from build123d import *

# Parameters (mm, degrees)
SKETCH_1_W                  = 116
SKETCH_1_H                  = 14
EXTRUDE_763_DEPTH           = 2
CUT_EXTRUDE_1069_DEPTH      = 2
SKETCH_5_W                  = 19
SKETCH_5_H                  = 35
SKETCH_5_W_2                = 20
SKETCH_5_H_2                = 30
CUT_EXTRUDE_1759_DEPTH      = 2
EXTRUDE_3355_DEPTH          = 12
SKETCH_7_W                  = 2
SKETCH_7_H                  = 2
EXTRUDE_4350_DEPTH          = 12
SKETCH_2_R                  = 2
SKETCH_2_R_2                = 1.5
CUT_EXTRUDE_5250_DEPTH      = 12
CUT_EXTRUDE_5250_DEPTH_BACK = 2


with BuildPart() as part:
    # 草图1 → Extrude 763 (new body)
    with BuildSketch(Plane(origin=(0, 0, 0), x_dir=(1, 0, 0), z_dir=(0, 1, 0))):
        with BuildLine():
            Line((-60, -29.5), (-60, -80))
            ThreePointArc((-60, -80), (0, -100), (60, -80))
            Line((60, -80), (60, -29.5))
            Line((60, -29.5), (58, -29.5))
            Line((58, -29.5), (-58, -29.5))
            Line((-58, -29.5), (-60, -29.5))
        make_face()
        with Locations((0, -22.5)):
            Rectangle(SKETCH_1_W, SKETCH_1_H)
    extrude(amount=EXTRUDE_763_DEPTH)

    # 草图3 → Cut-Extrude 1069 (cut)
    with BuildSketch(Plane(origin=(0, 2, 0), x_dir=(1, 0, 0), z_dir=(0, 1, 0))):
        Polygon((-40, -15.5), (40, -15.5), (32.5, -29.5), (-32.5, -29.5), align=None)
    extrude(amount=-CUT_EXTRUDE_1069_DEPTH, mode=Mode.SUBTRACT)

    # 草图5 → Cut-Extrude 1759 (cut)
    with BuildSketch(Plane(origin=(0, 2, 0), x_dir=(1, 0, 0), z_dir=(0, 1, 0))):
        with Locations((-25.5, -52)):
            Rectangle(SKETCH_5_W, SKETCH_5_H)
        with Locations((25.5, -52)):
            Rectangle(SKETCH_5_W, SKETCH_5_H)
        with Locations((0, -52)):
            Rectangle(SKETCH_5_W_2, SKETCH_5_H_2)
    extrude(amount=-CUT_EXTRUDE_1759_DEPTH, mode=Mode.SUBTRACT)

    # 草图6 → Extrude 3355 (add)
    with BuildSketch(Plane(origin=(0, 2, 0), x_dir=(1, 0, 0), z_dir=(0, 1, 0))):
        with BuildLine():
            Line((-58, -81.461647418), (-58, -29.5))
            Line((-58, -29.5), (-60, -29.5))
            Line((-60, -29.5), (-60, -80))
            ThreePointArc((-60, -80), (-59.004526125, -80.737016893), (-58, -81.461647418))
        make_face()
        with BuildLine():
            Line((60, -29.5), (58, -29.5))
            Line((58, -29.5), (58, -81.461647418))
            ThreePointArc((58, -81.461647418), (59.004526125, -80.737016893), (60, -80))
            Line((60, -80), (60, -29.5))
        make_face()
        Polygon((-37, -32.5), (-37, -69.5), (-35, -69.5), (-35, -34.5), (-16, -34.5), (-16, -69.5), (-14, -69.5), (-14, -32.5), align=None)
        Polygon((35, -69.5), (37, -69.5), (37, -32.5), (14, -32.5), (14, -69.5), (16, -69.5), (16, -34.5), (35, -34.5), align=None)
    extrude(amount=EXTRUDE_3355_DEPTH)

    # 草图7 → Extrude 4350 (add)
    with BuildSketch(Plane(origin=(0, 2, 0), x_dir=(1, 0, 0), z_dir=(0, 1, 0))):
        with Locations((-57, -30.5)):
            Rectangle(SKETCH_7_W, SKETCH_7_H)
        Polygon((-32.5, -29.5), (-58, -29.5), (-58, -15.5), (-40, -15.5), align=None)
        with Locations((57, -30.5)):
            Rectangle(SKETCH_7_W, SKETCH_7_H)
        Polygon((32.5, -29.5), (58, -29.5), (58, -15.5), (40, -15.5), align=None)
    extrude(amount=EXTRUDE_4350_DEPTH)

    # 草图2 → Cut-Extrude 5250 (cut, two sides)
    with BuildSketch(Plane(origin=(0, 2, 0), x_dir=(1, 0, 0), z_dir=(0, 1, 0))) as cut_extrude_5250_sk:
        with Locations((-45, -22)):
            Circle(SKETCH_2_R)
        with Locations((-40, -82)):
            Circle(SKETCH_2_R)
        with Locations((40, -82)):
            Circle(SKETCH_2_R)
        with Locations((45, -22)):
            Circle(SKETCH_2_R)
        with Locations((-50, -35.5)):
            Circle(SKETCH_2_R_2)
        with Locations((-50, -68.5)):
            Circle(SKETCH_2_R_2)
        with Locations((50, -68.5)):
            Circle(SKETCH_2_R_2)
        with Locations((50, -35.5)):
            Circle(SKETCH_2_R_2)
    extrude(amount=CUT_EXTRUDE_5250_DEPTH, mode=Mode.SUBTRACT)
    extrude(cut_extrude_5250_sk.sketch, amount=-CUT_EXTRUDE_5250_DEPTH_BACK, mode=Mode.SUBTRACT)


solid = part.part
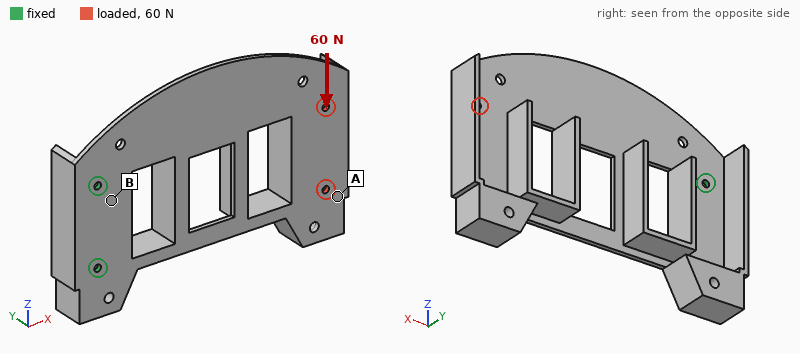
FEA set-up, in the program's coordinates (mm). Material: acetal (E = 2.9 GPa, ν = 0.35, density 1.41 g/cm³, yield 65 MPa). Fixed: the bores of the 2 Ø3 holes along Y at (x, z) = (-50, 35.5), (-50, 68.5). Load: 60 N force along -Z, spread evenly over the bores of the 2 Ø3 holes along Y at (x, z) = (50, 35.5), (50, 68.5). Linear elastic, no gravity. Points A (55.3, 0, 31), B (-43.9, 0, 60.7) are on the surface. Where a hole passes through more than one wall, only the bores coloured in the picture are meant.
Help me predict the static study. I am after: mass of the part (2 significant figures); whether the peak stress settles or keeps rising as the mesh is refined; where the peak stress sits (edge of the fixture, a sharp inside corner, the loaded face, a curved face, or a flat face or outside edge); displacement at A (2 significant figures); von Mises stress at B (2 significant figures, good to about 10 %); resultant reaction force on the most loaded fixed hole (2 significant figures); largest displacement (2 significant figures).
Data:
38 g
keeps rising
edge of the fixture
1.2 mm
5.7 MPa
180 N
1.5 mm
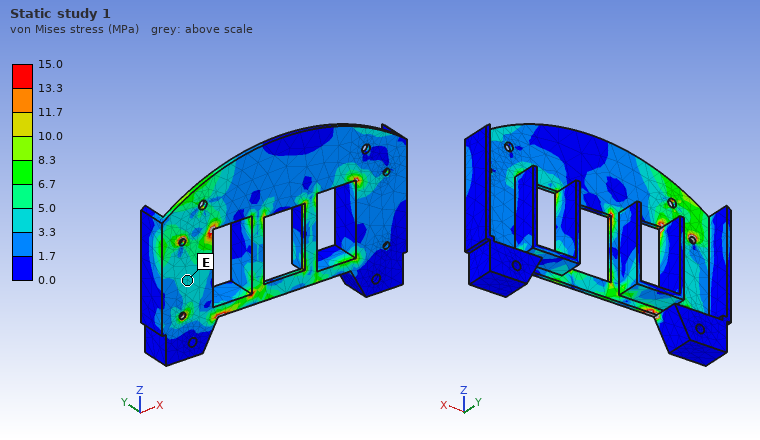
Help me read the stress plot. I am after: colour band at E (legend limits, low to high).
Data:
3.3 to 5.0 MPa
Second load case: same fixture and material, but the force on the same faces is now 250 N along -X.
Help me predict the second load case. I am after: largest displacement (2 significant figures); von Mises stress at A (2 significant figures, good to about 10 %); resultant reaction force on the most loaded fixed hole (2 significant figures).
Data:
0.93 mm
2.5 MPa
130 N
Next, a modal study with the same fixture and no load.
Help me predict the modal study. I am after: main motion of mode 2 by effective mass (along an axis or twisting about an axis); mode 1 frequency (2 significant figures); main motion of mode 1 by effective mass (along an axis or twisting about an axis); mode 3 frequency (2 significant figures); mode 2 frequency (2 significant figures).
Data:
twisting about X
26 Hz
along Y
200 Hz
84 Hz
